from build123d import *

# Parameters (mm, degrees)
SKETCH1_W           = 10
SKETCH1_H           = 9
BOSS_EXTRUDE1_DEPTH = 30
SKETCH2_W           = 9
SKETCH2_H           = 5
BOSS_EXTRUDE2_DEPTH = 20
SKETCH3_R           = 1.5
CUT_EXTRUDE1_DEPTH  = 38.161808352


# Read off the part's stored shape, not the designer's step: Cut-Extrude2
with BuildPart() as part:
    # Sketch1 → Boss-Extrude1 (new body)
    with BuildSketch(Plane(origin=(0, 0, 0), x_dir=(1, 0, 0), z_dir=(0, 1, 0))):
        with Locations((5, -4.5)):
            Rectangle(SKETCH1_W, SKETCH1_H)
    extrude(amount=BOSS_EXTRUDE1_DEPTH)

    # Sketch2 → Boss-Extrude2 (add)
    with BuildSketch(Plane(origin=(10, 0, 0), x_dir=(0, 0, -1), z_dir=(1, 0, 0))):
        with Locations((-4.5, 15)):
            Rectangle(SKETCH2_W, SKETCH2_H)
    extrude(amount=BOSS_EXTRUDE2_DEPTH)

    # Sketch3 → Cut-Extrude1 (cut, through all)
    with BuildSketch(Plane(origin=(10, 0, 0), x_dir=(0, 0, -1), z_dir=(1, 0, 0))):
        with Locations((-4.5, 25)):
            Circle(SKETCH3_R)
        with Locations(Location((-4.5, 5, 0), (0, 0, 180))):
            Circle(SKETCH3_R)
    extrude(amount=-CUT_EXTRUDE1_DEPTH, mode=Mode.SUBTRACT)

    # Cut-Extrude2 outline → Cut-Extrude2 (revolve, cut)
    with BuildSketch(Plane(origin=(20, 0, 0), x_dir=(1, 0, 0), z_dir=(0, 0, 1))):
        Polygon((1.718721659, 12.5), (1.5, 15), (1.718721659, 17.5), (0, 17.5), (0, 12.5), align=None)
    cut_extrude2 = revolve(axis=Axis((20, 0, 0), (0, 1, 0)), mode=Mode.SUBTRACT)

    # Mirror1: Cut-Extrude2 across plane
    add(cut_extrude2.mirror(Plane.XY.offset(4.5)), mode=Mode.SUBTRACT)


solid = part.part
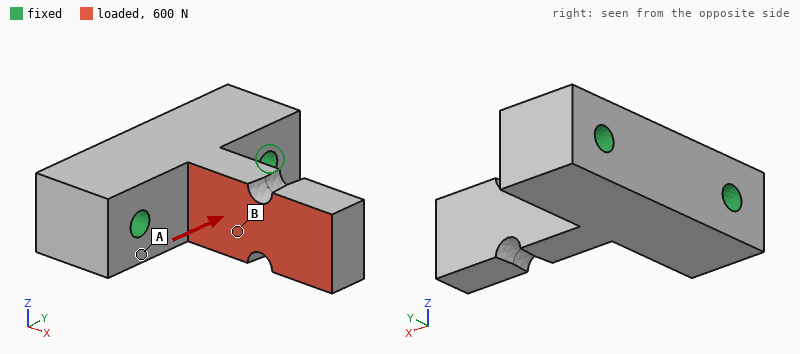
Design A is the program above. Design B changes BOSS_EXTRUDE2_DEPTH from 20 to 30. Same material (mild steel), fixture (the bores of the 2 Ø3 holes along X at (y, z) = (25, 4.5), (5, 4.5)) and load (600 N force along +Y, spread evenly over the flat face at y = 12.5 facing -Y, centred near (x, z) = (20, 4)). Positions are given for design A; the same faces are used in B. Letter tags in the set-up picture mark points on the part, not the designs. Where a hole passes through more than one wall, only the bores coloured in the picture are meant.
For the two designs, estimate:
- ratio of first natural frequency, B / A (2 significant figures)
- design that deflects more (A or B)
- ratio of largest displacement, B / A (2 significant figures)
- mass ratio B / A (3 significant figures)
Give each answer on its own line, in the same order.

0.46
B
3.1
1.13
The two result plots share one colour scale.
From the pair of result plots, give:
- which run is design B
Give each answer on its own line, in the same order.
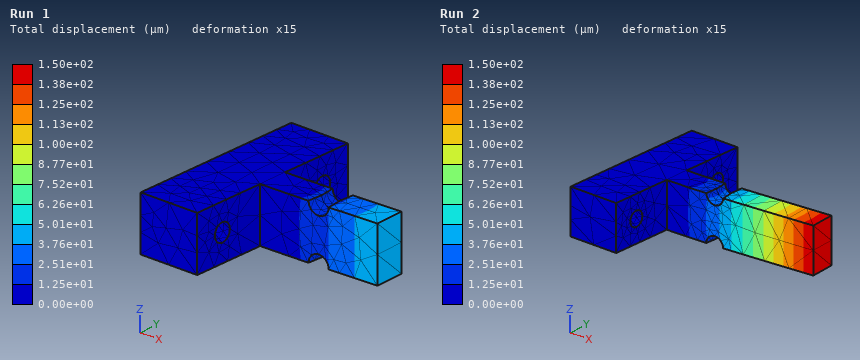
Run 2
